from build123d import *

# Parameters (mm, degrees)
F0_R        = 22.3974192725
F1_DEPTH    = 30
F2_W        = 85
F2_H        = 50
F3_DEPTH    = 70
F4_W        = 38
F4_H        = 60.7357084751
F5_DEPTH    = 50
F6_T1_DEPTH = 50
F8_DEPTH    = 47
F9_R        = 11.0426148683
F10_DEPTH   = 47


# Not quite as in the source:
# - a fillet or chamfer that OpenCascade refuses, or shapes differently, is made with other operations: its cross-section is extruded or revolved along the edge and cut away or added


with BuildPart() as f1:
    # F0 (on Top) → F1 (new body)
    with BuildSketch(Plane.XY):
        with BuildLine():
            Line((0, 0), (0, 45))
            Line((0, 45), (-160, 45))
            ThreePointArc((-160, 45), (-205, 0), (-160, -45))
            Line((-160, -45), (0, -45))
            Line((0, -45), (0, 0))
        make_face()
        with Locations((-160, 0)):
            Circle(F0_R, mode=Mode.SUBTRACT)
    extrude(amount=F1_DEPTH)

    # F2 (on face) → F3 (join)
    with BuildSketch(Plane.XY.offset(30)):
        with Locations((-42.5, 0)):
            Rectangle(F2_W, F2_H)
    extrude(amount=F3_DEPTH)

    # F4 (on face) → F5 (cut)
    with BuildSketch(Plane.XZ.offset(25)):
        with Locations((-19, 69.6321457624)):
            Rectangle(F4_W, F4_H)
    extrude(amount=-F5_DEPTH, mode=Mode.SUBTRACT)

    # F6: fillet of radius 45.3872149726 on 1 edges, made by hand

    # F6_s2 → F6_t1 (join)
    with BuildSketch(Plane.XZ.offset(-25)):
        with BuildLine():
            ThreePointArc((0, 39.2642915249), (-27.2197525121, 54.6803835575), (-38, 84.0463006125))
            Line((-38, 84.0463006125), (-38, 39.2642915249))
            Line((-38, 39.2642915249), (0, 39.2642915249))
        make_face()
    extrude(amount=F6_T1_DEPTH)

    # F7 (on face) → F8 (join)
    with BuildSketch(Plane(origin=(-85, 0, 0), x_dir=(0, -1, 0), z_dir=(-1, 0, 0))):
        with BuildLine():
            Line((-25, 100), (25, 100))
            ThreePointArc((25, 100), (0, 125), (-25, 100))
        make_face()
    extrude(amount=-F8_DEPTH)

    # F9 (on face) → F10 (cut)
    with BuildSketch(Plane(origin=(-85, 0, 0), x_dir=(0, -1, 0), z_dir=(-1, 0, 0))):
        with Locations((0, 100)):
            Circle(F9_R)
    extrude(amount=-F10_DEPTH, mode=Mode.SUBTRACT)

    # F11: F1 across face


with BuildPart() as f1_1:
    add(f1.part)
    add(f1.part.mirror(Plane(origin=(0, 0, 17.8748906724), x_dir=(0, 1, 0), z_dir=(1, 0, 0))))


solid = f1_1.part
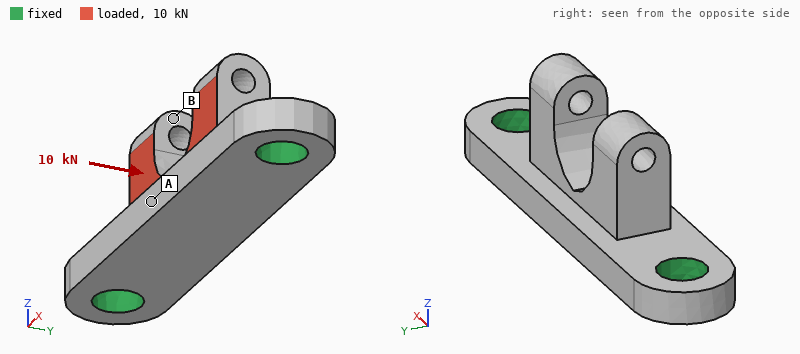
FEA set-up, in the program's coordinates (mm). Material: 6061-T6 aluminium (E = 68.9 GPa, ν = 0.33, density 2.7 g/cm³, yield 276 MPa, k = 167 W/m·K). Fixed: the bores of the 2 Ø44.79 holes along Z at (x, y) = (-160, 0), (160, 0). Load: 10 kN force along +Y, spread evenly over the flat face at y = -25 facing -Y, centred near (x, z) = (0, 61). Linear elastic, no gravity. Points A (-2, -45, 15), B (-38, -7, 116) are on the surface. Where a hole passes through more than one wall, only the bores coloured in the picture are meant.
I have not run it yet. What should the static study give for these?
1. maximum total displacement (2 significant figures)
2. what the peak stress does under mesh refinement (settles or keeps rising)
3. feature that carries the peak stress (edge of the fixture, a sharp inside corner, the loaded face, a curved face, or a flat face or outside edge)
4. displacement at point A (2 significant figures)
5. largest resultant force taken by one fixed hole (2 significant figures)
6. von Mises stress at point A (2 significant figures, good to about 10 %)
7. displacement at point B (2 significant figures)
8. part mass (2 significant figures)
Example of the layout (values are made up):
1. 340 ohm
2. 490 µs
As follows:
1. 0.11 mm
2. keeps rising
3. edge of the fixture
4. 0.041 mm
5. 5.0 kN
6. 4.3 MPa
7. 0.11 mm
8. 3.8 kg
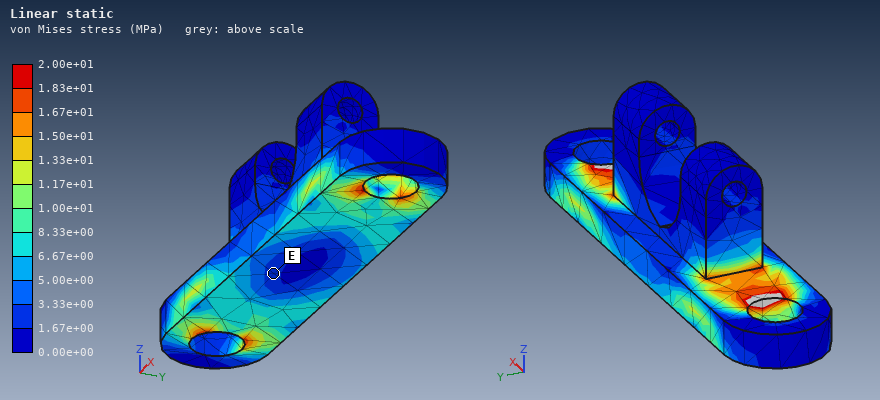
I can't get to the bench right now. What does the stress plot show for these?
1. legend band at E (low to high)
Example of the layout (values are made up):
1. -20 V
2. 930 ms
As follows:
1. 1.67e+00 to 3.33e+00 MPa
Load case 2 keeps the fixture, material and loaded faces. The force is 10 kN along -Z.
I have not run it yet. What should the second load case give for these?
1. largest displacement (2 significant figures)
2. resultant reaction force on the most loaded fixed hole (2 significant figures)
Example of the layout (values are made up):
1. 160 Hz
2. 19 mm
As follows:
1. 74 µm
2. 5.6 kN
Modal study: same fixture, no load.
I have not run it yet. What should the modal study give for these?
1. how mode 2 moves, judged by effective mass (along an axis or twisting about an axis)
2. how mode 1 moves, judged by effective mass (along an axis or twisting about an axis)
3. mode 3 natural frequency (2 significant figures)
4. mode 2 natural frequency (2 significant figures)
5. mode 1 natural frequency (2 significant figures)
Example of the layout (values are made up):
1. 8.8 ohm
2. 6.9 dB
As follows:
1. along Z
2. along Y
3. 2800 Hz
4. 1600 Hz
5. 1400 Hz
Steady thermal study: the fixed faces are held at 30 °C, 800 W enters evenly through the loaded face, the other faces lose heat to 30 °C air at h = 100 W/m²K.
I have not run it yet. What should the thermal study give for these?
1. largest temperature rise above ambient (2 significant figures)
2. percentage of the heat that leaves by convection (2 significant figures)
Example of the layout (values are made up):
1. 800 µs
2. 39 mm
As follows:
1. 67 K
2. 47 %
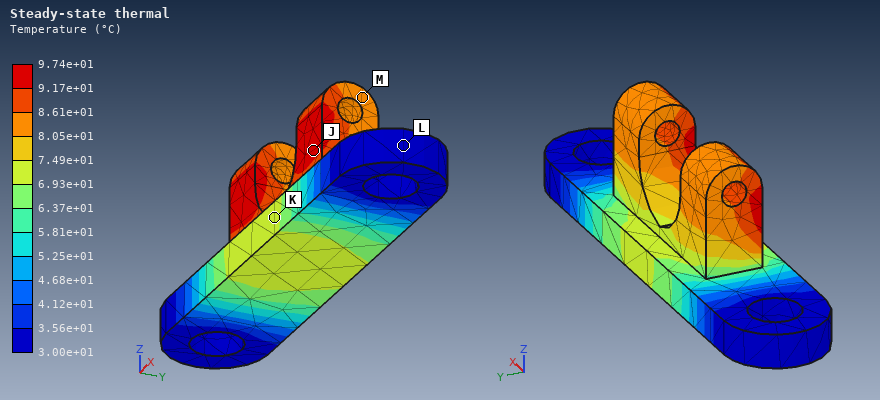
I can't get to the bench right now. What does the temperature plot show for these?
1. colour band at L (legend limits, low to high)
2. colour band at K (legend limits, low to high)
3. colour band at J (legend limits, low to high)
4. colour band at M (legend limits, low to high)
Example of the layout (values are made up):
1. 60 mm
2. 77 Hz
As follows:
1. 3.00e+01 to 3.56e+01 °C
2. 6.93e+01 to 7.49e+01 °C
3. 9.17e+01 to 9.74e+01 °C
4. 8.05e+01 to 8.61e+01 °C
